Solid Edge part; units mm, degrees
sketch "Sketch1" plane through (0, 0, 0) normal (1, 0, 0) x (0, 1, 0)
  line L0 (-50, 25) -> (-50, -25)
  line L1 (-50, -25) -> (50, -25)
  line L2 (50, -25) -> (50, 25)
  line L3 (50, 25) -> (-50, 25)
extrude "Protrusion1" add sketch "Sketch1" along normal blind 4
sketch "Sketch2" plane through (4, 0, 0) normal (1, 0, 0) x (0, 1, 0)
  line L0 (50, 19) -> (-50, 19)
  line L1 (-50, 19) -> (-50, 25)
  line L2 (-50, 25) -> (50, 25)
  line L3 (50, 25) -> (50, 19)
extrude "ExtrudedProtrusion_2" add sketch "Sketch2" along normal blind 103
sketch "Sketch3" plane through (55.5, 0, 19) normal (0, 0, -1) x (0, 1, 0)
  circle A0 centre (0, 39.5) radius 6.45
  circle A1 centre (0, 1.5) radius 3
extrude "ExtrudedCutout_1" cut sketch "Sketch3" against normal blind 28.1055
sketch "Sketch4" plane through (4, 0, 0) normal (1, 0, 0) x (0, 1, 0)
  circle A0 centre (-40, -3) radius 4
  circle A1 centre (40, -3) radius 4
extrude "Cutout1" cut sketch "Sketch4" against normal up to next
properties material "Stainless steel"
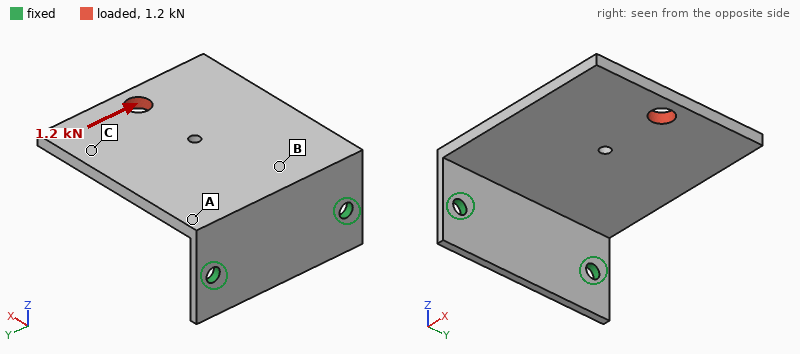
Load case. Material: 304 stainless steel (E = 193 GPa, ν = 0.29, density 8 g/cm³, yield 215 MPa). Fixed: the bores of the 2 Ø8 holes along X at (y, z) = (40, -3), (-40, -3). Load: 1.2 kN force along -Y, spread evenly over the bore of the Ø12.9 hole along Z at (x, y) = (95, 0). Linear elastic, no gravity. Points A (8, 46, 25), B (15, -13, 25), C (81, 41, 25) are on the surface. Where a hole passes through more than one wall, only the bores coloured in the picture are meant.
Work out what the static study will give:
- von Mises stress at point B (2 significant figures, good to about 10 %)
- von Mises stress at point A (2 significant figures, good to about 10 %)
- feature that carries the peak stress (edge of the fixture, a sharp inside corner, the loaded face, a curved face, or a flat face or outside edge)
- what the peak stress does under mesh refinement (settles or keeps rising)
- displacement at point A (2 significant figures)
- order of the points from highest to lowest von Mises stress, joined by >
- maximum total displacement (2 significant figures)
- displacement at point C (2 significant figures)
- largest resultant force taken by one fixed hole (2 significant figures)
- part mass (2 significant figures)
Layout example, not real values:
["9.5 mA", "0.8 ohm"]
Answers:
["32 MPa", "62 MPa", "edge of the fixture", "keeps rising", "0.097 mm", "A > B > C", "0.25 mm", "0.19 mm", "1.6 kN", "640 g"]
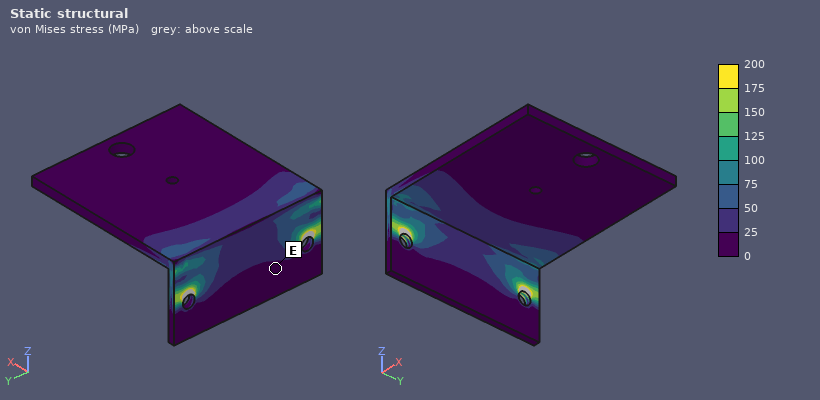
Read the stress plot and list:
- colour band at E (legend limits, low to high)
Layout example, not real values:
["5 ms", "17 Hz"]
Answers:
["0 to 25 MPa"]
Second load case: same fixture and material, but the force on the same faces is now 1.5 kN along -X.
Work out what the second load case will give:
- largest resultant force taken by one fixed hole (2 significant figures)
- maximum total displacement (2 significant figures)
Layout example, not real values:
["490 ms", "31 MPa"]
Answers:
["750 N", "0.52 mm"]
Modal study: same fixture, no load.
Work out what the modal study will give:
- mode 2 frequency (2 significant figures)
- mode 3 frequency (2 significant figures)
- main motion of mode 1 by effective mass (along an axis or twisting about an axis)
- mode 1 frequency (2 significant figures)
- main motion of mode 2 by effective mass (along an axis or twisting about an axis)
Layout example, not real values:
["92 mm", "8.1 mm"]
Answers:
["730 Hz", "1100 Hz", "along Z", "210 Hz", "along Y"]
